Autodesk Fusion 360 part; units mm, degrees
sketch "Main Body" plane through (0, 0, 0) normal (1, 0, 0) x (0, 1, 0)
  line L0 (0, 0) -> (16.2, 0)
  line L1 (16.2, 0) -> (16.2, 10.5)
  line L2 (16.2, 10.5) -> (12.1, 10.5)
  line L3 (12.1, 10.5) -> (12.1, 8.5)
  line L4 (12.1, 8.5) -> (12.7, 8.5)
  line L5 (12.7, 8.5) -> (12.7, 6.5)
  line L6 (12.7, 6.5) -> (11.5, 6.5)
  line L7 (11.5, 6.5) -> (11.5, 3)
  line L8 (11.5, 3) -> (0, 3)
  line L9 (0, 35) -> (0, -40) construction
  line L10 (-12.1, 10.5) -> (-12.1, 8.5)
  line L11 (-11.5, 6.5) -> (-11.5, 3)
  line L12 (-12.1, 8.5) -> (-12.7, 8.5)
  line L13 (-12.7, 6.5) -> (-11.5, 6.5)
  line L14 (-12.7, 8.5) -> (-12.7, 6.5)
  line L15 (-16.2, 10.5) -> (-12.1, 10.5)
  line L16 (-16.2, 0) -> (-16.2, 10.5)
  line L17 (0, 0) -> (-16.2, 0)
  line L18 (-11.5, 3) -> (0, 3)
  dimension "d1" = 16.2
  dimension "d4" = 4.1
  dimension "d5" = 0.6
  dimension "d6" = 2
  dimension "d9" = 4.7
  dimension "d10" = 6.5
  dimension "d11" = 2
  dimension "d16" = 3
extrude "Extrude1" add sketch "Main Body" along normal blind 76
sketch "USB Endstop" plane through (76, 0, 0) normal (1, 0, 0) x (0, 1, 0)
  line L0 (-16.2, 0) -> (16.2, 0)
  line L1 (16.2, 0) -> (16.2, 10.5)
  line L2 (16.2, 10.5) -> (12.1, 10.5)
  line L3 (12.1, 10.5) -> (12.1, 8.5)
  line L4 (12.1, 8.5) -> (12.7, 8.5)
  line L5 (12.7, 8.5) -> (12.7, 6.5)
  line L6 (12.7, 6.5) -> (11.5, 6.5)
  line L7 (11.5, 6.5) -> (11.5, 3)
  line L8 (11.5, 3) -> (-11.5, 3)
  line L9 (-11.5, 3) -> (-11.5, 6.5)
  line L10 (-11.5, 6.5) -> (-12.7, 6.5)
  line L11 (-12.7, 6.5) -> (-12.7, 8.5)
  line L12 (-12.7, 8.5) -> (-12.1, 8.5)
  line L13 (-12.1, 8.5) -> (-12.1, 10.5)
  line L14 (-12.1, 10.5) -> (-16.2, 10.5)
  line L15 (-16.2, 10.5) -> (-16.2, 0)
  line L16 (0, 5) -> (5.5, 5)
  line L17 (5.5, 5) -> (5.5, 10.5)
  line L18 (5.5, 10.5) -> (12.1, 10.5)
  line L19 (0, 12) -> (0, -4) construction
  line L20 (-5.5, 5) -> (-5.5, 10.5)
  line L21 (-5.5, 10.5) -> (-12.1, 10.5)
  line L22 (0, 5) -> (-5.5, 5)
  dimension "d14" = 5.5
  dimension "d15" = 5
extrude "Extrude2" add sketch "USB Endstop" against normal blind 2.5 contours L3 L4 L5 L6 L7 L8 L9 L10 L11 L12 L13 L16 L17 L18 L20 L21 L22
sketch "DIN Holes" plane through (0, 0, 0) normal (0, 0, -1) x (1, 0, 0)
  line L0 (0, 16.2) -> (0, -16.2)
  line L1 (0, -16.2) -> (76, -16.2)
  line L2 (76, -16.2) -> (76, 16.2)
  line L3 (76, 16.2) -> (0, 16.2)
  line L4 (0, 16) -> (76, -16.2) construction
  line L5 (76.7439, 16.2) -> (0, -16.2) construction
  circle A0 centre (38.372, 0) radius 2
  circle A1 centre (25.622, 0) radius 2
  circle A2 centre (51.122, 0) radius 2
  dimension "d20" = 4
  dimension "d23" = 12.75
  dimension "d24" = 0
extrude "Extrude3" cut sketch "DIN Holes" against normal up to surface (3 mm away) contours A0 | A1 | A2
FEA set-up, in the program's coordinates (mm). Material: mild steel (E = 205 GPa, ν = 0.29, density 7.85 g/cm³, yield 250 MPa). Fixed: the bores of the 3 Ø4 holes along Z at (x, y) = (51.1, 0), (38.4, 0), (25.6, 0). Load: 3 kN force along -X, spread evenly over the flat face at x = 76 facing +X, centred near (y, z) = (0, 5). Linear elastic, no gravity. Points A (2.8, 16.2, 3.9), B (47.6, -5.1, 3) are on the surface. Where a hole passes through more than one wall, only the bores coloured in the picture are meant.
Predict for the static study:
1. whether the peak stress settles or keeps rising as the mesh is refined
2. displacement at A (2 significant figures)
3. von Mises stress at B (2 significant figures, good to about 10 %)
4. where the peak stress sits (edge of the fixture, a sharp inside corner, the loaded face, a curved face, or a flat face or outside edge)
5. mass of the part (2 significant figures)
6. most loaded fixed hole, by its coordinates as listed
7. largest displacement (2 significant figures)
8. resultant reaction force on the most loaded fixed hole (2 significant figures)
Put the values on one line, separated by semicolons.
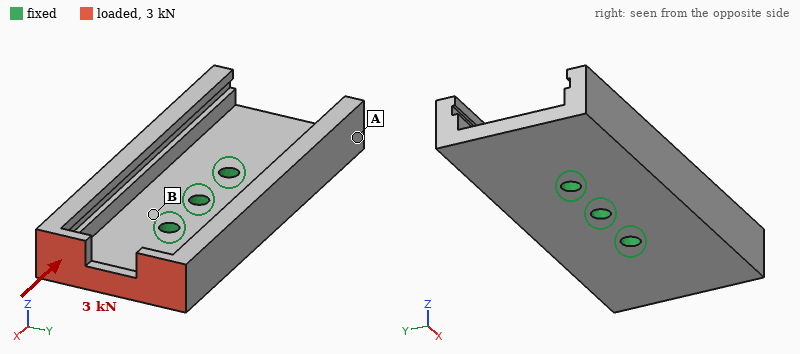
keeps rising; 12 µm; 33 MPa; edge of the fixture; 97 g; (51.1, 0); 31 µm; 1.6 kN
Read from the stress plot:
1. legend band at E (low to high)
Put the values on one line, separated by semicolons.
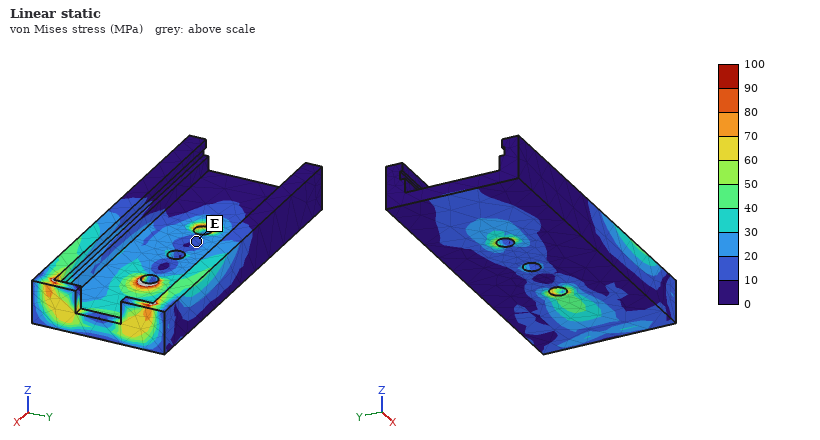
10 to 20 MPa
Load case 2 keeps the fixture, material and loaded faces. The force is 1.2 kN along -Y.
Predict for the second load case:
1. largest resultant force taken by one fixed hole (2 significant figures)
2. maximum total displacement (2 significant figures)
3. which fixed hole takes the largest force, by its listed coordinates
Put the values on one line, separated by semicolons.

2.3 kN; 49 µm; (51.1, 0)
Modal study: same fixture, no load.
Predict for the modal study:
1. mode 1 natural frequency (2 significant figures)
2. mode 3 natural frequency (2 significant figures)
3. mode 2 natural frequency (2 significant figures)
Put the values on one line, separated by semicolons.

3800 Hz; 4200 Hz; 4000 Hz
